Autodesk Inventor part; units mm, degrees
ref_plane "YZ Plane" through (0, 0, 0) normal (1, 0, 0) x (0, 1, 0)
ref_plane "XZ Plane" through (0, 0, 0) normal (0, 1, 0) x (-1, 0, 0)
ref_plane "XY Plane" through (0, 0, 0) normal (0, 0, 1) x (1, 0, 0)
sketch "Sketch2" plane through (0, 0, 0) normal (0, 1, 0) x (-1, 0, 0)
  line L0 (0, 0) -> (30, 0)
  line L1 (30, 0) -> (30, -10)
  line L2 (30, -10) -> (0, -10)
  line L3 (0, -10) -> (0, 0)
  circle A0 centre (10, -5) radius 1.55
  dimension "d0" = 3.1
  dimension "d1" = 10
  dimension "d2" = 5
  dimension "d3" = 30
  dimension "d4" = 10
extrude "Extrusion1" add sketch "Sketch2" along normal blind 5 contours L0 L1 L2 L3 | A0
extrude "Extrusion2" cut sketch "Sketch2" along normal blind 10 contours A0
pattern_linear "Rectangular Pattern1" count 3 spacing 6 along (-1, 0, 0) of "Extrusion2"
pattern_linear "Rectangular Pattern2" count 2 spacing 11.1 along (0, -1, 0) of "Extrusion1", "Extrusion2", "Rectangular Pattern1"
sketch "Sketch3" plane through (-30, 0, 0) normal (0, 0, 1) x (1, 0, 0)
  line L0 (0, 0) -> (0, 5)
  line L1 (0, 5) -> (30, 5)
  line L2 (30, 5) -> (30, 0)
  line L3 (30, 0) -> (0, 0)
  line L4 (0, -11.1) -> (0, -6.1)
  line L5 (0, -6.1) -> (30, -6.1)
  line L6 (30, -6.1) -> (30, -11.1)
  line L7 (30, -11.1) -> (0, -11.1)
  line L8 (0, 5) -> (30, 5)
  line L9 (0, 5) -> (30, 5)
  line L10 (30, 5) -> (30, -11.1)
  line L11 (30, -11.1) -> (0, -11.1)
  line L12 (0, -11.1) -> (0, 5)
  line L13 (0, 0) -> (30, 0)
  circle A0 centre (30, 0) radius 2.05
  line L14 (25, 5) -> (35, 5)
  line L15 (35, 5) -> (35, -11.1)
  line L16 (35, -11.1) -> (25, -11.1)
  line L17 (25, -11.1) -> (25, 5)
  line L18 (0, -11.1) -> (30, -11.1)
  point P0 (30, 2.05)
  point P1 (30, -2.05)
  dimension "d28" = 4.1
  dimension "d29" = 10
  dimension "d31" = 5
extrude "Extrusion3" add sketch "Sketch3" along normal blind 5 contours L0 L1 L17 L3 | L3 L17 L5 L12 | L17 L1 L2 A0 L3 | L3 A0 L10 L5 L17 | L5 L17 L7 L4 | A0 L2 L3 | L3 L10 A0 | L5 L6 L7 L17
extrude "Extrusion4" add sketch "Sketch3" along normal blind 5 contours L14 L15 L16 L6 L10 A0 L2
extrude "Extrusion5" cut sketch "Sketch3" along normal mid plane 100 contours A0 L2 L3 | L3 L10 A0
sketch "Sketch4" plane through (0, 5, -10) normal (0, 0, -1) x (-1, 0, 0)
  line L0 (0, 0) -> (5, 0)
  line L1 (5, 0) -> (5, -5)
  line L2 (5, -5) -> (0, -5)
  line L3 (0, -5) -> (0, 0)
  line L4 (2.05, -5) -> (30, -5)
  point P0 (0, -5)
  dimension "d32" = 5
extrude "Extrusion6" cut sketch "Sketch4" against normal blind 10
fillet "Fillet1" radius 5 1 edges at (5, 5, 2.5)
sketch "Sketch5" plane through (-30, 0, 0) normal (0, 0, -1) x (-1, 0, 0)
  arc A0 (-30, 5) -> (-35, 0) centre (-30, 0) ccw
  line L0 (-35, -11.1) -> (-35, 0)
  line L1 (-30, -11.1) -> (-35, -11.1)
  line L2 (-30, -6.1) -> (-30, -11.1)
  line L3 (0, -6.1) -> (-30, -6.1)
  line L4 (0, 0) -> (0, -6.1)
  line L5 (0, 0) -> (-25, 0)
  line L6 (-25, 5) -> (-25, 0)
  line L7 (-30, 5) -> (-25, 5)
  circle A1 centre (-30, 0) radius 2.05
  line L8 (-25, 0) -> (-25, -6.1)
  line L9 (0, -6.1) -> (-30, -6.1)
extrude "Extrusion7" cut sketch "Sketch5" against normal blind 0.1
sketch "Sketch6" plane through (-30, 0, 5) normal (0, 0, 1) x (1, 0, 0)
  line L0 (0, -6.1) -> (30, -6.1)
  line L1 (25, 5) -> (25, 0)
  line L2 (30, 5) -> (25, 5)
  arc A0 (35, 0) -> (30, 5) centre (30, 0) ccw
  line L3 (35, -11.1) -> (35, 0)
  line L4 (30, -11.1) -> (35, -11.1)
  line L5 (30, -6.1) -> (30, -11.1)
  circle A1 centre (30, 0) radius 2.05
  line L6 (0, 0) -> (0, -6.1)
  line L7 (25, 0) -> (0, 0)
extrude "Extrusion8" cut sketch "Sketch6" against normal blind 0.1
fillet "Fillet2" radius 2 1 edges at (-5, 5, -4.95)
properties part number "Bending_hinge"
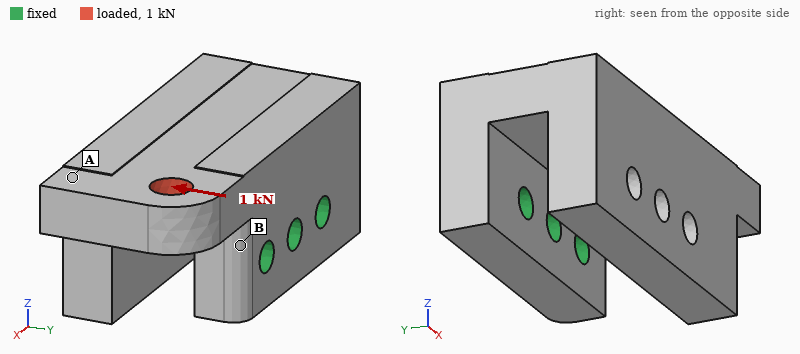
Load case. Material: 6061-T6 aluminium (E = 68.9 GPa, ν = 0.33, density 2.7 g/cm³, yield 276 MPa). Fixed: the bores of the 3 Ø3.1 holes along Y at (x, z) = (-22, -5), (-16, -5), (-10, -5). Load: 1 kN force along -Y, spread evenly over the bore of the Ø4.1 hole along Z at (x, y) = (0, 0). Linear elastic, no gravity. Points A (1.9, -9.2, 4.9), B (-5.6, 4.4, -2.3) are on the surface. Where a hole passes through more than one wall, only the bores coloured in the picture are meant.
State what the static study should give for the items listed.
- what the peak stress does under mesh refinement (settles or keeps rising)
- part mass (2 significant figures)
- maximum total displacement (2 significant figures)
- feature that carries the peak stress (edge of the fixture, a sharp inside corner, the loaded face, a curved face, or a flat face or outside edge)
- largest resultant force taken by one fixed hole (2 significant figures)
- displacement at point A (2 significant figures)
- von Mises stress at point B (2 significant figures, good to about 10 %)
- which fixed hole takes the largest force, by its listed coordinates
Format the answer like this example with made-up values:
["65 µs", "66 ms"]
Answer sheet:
["keeps rising", "14 g", "78 µm", "edge of the fixture", "1.3 kN", "67 µm", "72 MPa", "(-10, -5)"]
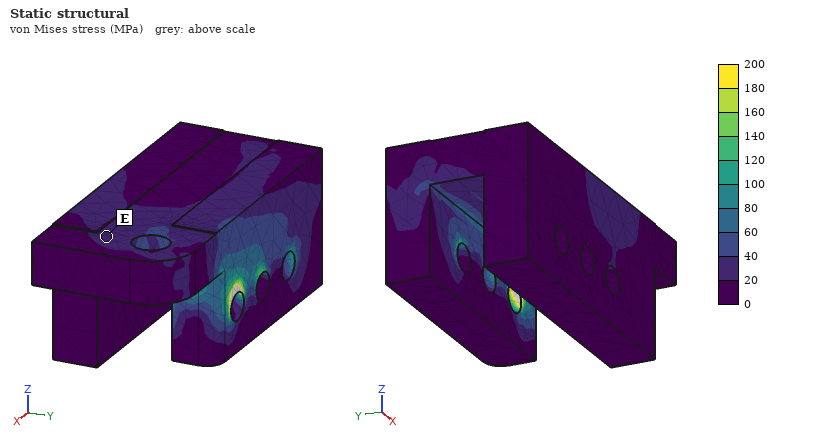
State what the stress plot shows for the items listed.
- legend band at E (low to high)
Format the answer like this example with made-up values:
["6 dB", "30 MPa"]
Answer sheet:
["20 to 40 MPa"]
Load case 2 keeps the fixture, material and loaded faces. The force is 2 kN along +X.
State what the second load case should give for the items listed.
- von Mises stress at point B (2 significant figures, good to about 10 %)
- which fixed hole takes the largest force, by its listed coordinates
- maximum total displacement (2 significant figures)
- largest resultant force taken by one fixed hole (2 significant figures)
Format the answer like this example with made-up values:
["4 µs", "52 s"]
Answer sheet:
["32 MPa", "(-10, -5)", "23 µm", "1.3 kN"]
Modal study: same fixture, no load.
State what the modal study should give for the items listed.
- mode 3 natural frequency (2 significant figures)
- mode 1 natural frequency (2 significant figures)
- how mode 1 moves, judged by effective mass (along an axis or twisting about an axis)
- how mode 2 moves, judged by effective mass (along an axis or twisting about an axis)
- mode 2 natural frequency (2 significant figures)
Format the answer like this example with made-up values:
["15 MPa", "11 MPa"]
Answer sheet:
["13 kHz", "6600 Hz", "along Z", "along X", "8900 Hz"]
